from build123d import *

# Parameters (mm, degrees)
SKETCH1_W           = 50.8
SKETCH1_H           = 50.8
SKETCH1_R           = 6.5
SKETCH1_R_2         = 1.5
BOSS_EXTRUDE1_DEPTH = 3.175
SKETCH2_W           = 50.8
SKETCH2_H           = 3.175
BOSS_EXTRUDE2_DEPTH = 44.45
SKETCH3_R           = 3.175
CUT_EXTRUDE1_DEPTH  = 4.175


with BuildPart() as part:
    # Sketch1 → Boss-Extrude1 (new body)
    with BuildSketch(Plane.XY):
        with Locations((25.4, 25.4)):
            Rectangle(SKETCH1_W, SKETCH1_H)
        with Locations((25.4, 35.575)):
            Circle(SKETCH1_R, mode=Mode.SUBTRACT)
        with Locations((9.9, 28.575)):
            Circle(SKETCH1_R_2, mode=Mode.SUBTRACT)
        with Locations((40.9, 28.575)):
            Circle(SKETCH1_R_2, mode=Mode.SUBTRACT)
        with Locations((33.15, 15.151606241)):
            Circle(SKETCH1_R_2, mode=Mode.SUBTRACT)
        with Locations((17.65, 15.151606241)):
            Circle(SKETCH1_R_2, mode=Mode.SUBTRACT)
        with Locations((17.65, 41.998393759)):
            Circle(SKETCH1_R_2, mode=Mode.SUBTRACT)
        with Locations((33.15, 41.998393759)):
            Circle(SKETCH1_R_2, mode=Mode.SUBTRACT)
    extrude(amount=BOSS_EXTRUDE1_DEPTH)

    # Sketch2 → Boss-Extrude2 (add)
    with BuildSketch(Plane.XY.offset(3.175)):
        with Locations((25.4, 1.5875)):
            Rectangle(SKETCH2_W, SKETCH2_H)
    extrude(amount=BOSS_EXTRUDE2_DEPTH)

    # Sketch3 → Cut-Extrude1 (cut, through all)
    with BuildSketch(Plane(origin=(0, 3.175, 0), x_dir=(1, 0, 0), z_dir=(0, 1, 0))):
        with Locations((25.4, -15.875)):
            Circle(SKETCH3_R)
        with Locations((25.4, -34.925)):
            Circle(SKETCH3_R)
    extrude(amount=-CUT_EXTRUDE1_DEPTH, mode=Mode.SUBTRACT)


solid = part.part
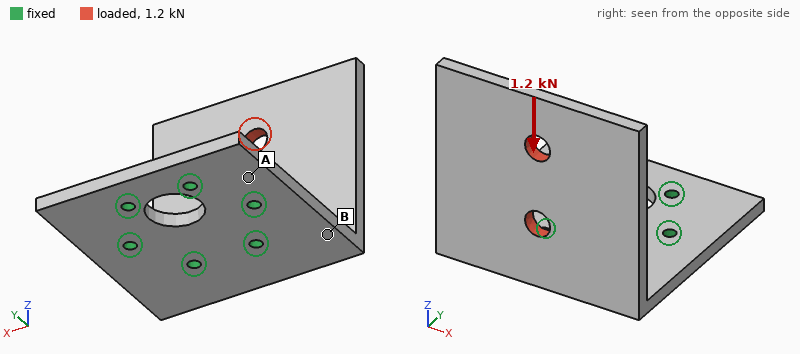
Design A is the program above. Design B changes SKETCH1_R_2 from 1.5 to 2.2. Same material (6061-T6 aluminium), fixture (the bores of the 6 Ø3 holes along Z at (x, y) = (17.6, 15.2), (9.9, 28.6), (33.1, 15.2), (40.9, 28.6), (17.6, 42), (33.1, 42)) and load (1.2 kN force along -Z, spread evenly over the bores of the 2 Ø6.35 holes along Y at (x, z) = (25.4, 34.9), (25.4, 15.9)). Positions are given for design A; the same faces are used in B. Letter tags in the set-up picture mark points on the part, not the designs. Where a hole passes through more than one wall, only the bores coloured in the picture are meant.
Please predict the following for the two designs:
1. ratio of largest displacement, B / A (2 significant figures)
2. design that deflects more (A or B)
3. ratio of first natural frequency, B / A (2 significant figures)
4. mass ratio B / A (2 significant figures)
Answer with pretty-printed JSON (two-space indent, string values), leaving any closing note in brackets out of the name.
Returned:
{
  "ratio of largest displacement, B / A": "0.87",
  "design that deflects more": "A",
  "ratio of first natural frequency, B / A": "1.0",
  "mass ratio B / A": "0.99"
}
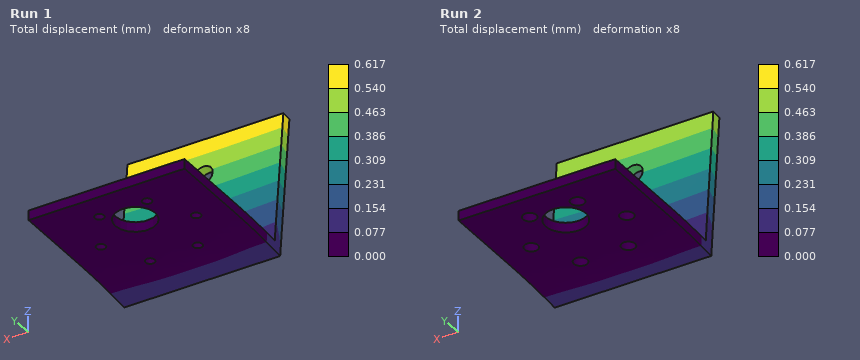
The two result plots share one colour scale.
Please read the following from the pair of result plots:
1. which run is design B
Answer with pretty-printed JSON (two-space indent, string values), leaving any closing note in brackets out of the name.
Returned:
{
  "which run is design B": "Run 2"
}
